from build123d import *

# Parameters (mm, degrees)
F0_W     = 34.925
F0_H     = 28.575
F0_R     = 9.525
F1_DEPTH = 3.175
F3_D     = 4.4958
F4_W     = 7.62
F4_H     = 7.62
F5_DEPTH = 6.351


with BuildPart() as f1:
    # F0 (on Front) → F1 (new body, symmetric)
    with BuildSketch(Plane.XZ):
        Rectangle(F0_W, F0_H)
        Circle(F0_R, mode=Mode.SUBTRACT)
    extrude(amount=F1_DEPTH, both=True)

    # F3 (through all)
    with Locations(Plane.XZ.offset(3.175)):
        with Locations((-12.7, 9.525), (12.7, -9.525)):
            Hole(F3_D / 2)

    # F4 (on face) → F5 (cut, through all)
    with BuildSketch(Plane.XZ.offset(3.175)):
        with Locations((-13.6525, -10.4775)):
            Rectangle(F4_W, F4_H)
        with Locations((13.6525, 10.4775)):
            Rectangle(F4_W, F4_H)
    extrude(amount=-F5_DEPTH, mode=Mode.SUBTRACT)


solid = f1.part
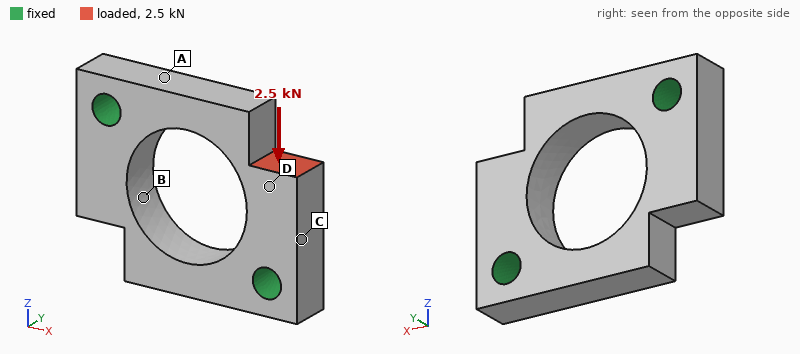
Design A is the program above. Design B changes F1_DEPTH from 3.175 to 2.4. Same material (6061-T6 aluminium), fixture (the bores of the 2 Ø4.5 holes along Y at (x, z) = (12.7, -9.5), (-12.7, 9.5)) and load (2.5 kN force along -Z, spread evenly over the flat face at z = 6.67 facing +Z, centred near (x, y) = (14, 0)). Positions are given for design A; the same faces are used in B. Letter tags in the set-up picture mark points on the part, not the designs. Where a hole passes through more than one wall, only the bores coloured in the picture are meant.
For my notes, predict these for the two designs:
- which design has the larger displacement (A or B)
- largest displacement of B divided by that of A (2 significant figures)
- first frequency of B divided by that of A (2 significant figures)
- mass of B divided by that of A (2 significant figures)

B
1.3
0.81
0.76
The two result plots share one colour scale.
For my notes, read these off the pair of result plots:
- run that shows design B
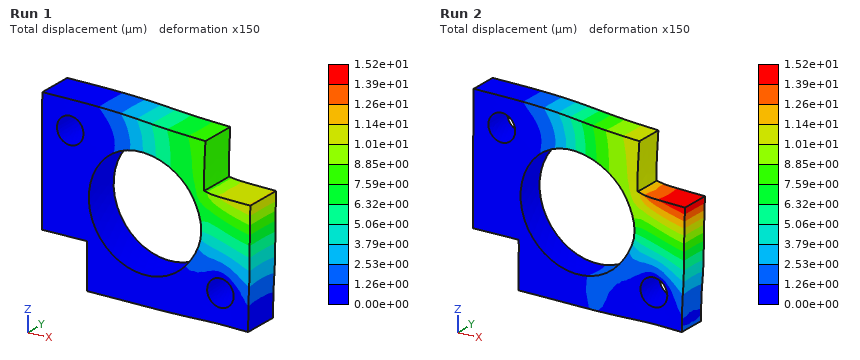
Run 2
